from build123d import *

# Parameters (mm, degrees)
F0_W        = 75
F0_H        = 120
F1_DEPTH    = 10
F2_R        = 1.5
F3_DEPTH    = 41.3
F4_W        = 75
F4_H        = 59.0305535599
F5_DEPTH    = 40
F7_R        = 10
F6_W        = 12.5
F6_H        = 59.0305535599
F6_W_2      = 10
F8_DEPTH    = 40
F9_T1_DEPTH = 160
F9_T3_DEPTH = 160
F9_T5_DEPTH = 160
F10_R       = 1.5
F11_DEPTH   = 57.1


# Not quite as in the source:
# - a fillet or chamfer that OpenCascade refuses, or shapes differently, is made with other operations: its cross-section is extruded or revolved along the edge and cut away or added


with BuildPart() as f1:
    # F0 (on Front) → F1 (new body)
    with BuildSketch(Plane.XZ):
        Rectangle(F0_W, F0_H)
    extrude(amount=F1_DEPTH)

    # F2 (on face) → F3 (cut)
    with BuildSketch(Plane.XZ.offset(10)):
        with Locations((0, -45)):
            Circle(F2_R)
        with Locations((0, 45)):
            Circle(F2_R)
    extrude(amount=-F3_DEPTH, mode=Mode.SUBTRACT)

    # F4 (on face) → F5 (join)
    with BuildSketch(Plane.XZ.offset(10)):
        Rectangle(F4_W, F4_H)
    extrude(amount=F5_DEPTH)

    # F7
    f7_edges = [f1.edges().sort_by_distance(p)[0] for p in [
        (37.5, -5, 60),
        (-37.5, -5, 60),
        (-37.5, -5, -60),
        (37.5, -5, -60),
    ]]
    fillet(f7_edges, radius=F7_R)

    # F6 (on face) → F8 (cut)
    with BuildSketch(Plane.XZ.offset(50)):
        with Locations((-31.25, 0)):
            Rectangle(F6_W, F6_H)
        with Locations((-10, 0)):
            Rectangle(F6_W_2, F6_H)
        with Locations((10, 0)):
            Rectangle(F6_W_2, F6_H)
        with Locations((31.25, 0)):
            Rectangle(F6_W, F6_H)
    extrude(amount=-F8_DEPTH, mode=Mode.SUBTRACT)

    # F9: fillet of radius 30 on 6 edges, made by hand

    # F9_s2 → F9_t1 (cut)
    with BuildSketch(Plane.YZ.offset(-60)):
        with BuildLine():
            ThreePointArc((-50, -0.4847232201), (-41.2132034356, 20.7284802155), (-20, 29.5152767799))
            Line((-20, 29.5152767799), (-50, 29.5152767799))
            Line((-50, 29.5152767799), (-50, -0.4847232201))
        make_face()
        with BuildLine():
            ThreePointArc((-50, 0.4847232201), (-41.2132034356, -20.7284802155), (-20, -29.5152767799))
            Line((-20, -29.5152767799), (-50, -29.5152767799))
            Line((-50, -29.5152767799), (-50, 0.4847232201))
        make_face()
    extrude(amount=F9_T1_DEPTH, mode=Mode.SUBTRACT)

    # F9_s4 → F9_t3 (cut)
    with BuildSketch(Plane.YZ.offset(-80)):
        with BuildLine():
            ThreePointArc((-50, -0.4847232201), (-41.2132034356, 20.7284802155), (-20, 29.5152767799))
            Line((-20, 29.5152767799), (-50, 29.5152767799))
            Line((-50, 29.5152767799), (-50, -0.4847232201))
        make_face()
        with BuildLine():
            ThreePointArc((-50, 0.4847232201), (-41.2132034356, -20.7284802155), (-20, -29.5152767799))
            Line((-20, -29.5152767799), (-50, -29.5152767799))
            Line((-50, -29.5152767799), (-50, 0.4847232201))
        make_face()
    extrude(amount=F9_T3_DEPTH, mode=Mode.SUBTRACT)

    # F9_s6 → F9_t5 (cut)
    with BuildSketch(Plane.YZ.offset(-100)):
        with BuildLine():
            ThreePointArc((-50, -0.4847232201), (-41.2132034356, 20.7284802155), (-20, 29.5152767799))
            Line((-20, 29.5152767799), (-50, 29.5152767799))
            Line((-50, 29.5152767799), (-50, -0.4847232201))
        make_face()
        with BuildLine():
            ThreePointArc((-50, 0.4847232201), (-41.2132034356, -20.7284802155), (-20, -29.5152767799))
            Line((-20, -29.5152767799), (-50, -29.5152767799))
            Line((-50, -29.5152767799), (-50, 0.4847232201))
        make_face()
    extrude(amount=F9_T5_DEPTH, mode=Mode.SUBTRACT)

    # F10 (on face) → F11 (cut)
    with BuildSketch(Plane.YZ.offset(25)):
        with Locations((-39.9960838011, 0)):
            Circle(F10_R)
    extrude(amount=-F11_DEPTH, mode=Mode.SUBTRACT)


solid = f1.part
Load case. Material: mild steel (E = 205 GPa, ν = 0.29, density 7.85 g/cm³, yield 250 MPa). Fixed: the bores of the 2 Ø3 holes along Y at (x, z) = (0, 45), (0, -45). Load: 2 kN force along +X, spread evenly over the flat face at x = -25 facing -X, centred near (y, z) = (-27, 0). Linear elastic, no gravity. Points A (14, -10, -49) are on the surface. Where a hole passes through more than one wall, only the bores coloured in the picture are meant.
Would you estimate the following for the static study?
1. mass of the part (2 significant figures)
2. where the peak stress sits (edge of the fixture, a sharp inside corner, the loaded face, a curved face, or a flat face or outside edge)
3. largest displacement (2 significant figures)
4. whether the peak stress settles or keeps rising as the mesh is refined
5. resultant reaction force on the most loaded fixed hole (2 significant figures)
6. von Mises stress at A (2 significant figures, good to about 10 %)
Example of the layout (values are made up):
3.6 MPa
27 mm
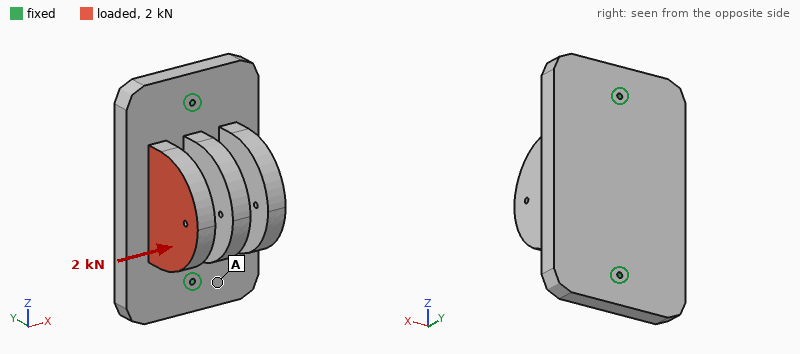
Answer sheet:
1.2 kg
edge of the fixture
60 µm
keeps rising
1.0 kN
8.2 MPa
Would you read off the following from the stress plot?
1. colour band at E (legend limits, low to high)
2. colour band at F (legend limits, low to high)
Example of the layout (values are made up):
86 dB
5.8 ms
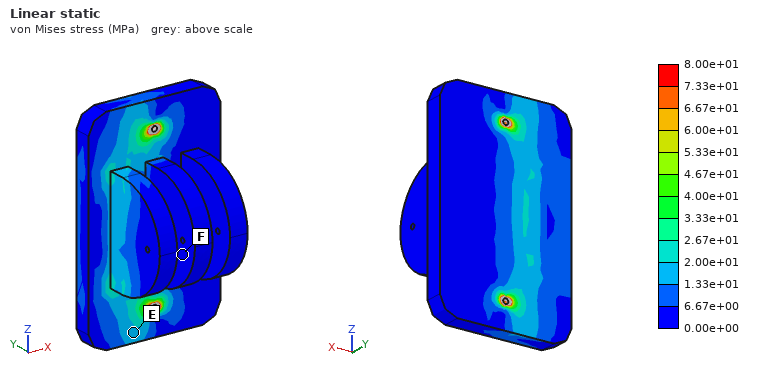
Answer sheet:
1.33e+01 to 2.00e+01 MPa
0.00e+00 to 6.67e+00 MPa
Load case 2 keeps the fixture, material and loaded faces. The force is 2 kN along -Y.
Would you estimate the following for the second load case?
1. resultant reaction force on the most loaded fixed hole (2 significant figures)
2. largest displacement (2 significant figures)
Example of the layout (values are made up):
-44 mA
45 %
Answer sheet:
1.0 kN
47 µm
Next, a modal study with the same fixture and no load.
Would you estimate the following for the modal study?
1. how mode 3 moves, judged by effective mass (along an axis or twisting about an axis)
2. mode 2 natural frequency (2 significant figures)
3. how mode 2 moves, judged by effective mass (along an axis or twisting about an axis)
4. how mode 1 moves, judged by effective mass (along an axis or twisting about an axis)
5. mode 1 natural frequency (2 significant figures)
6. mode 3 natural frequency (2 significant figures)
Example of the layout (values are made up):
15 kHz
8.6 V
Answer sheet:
along Y
3200 Hz
along Y
along X
1700 Hz
4500 Hz
